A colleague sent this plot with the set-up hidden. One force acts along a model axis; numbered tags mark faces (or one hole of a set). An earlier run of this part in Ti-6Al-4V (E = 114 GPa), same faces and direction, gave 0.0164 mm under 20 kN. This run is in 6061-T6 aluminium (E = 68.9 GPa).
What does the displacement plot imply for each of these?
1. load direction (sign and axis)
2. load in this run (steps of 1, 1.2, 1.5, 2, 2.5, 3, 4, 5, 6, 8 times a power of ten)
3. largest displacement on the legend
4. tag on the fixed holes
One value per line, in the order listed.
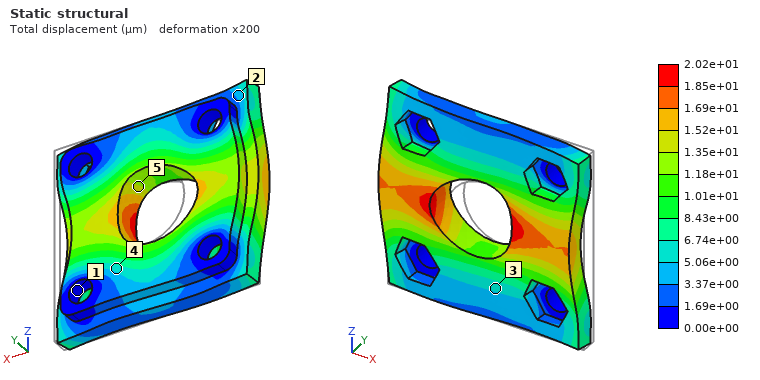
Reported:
-X
15 kN
2.02e+01 µm
1
